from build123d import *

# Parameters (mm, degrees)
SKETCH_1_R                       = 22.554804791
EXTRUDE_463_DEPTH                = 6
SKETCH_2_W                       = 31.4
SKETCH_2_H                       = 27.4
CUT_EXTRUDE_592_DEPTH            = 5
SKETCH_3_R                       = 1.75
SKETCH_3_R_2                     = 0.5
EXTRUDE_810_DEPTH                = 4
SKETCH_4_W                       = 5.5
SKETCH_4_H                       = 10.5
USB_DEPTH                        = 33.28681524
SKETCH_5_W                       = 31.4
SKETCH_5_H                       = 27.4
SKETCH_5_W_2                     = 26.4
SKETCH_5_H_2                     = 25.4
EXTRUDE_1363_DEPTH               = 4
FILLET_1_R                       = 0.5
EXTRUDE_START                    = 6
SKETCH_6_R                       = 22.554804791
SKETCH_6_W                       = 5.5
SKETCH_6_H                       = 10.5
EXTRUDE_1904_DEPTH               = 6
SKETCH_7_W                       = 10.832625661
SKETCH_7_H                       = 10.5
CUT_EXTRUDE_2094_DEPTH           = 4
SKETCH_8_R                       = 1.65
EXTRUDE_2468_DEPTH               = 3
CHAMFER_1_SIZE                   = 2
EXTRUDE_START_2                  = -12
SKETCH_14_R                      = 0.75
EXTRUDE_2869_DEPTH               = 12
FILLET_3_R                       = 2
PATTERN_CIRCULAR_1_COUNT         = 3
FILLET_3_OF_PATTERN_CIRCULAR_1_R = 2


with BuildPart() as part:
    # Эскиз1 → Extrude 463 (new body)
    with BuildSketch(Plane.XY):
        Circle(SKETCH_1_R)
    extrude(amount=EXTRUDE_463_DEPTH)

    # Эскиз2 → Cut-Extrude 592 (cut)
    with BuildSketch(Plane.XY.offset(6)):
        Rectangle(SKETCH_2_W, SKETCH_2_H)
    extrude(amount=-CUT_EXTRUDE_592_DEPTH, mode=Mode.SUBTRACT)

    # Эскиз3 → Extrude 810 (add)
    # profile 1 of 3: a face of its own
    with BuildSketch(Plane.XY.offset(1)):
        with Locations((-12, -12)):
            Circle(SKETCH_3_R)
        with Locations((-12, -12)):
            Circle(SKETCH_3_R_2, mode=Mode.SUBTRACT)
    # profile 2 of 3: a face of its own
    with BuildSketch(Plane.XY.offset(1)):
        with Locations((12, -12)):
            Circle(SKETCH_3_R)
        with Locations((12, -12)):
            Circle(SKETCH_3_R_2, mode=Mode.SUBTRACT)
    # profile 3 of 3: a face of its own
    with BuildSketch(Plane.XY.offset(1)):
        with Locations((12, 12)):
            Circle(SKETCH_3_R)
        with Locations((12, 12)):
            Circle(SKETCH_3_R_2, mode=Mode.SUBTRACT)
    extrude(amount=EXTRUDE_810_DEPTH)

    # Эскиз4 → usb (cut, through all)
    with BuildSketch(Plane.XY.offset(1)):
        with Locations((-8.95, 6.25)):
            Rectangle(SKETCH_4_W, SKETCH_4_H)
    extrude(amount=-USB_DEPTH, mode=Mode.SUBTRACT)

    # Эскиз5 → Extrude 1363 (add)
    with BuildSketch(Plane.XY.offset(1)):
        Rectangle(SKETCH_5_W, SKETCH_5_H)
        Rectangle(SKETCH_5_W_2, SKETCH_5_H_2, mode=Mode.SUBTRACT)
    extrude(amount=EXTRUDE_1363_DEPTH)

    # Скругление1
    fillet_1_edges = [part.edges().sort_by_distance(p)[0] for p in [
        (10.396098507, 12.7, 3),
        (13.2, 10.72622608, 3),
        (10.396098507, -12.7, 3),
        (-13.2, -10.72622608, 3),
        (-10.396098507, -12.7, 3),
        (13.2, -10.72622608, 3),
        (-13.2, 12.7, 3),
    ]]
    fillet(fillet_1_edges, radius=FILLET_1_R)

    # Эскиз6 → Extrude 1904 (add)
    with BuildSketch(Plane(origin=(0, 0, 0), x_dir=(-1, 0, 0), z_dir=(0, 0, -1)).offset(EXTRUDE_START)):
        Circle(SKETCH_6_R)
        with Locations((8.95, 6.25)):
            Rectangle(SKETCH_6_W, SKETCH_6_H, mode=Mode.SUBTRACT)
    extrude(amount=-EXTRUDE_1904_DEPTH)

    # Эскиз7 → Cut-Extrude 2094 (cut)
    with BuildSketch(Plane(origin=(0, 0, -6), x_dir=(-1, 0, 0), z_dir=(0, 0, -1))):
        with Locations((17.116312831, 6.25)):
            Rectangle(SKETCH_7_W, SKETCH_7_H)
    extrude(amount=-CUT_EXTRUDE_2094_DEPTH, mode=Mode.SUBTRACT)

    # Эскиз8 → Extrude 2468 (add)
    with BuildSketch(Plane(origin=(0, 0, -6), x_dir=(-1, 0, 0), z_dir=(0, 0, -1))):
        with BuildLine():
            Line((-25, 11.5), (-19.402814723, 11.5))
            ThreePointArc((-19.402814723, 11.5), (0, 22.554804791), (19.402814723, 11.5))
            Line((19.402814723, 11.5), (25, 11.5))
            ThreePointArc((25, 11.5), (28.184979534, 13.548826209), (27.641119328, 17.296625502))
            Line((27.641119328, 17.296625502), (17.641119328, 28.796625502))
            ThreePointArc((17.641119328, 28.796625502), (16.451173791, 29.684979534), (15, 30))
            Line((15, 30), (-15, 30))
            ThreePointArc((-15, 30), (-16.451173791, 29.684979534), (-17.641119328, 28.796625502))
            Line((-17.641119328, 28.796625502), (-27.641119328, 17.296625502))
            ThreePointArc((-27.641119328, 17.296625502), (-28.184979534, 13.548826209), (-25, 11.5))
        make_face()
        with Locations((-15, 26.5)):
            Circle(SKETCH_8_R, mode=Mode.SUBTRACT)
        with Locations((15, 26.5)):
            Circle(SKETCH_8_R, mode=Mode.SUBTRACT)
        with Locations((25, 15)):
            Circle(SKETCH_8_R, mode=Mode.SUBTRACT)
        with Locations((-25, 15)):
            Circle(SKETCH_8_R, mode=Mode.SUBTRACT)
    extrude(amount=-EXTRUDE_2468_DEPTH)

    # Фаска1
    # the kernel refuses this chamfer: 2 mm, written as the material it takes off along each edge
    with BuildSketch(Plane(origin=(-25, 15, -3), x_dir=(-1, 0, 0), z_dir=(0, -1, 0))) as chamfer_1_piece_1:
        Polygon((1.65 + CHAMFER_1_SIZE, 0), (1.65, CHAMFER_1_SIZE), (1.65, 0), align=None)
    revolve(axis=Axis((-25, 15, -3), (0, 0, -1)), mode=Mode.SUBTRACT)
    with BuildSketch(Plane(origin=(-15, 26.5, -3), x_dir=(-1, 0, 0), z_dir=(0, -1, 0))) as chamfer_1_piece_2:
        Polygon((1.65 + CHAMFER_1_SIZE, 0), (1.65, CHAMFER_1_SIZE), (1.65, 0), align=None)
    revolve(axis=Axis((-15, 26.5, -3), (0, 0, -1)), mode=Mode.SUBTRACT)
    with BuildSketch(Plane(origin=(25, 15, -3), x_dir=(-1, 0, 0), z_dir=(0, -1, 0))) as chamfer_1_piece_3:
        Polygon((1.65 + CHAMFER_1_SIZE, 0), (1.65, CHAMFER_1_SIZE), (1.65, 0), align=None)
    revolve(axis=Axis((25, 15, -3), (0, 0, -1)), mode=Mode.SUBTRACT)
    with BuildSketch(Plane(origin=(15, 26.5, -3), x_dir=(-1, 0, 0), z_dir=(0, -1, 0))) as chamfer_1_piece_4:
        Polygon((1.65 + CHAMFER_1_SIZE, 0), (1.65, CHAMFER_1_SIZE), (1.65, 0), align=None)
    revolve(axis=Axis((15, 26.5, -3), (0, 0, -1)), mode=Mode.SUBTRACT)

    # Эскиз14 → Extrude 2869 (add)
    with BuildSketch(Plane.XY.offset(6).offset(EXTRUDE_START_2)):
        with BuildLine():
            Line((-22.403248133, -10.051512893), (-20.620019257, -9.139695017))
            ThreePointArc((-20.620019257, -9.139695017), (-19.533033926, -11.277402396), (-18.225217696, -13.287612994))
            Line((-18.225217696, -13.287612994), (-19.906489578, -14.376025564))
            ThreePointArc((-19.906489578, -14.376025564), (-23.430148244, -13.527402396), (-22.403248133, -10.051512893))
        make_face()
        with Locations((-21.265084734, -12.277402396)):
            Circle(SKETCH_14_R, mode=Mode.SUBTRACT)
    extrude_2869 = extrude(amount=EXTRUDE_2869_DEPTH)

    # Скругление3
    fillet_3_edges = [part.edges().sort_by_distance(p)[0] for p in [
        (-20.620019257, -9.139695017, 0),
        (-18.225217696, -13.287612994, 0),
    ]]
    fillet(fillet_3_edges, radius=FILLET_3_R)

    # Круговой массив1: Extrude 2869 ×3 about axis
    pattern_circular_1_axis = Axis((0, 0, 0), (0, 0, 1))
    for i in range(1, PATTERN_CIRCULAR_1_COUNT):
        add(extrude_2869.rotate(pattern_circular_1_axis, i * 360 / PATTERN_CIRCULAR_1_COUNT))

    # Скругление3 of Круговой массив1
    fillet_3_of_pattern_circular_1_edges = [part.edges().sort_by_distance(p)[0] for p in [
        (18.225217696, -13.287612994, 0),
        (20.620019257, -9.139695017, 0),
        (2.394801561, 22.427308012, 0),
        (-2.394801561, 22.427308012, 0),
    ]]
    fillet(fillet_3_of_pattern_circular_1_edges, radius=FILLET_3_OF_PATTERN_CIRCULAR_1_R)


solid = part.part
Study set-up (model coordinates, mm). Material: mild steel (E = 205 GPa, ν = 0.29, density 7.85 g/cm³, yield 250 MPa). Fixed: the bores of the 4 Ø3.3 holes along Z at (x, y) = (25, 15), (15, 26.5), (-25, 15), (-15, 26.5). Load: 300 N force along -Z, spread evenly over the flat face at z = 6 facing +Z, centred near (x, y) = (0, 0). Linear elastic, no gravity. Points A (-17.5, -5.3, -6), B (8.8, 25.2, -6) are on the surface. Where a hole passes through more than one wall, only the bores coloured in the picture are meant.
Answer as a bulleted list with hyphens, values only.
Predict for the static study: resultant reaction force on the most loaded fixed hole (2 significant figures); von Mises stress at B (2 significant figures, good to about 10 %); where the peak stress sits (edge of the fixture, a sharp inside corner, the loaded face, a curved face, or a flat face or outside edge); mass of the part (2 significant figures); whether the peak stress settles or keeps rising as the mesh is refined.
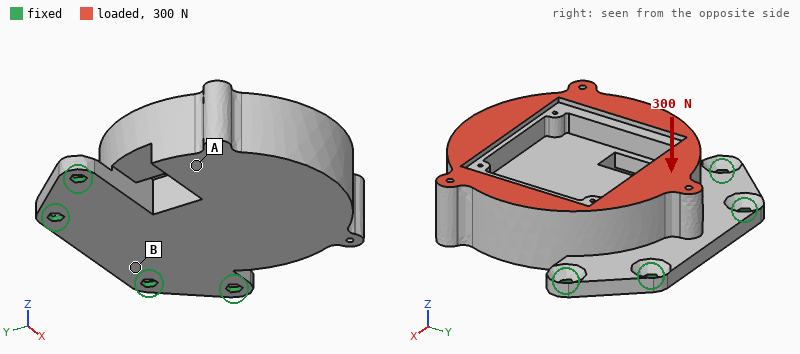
- 470 N
- 23 MPa
- edge of the fixture
- 130 g
- keeps rising
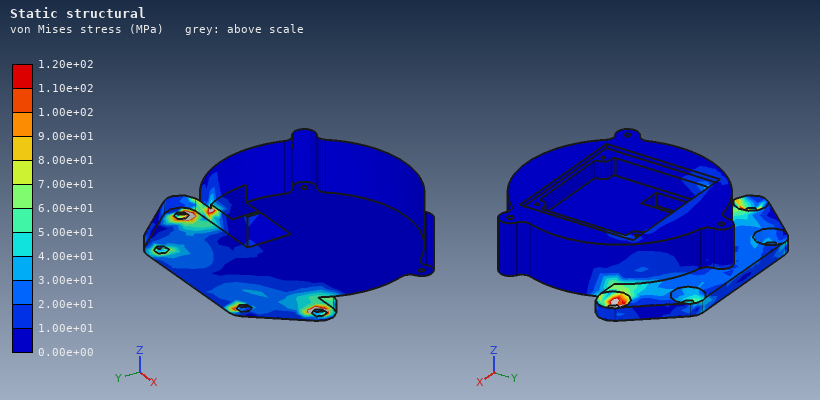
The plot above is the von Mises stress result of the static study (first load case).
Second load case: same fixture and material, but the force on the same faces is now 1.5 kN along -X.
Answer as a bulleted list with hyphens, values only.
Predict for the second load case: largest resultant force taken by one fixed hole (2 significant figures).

- 720 N
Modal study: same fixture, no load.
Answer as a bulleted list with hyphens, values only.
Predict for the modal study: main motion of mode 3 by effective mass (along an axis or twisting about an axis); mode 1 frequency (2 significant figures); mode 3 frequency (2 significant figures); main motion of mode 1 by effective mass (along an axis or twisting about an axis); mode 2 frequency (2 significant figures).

- along X
- 1300 Hz
- 6600 Hz
- along Z
- 5700 Hz
